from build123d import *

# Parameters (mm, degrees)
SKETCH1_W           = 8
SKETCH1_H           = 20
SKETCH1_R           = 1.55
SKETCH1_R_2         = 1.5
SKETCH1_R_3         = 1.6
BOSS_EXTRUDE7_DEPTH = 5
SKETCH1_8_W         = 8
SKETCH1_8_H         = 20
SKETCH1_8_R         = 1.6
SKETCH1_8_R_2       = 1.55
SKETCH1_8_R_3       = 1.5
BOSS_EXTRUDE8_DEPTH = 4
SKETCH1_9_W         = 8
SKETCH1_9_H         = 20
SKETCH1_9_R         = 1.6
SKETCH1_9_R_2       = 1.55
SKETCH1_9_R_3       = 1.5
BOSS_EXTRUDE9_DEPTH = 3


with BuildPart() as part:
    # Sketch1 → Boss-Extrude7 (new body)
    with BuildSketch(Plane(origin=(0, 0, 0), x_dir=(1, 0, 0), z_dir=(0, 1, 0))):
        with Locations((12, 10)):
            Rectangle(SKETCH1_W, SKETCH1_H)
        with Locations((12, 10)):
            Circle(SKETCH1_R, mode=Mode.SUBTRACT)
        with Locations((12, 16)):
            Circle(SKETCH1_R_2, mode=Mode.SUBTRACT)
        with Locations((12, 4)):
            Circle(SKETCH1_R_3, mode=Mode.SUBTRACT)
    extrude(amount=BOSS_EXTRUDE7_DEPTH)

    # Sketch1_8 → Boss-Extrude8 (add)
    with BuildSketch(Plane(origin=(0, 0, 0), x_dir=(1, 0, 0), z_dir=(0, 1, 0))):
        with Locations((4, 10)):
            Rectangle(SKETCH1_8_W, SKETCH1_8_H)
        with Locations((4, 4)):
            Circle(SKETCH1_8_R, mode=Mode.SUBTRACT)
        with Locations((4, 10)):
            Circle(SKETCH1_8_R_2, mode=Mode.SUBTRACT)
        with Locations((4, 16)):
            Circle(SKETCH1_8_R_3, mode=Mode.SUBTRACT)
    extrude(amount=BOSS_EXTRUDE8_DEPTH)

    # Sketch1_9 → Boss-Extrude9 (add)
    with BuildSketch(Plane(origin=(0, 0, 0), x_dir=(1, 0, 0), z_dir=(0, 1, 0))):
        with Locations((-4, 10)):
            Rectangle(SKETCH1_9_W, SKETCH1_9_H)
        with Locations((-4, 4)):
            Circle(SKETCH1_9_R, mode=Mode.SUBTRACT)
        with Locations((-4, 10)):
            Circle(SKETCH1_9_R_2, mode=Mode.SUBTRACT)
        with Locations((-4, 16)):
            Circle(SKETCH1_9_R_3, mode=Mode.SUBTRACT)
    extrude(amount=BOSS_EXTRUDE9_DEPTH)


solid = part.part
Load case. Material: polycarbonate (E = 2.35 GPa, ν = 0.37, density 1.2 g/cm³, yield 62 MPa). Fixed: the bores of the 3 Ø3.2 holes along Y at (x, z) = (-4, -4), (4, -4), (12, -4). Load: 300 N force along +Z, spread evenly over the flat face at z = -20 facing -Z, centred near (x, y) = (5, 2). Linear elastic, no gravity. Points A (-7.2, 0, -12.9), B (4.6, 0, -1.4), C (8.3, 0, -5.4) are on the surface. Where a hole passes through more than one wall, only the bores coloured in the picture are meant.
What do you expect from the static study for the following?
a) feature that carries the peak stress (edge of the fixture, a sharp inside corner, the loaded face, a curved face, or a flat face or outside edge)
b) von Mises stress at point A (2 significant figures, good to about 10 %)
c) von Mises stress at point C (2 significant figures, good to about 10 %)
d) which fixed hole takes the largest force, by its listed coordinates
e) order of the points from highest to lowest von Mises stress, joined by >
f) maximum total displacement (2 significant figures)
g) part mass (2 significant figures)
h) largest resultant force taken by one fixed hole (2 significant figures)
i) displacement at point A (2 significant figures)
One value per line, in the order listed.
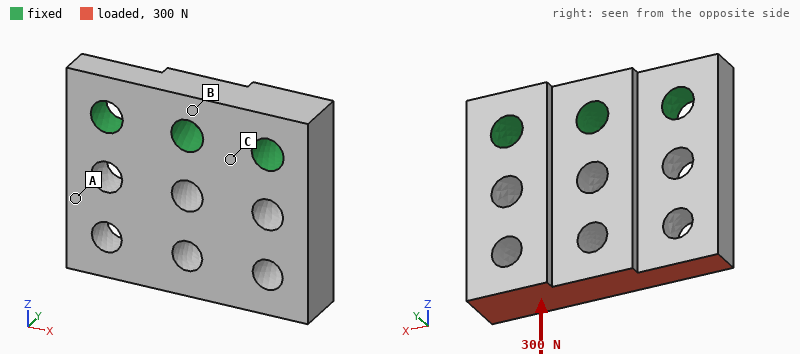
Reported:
a curved face
4.2 MPa
1.8 MPa
(12, -4)
A > C > B
32 µm
2.0 g
130 N
18 µm
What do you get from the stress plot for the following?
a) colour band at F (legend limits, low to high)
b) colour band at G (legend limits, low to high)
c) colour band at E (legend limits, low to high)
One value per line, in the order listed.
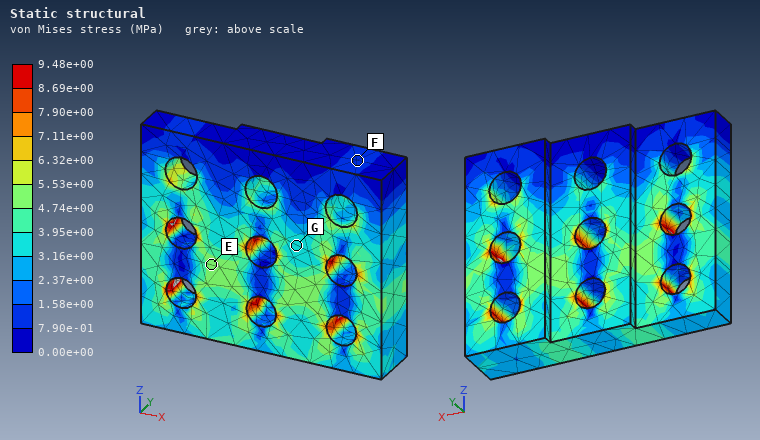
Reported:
7.90e-01 to 1.58e+00 MPa
3.16e+00 to 3.95e+00 MPa
4.74e+00 to 5.53e+00 MPa
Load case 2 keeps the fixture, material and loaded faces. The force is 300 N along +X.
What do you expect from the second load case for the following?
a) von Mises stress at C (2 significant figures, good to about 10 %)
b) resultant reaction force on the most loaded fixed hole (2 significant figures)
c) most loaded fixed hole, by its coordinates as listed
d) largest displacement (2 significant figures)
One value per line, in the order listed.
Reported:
3.9 MPa
300 N
(12, -4)
0.20 mm
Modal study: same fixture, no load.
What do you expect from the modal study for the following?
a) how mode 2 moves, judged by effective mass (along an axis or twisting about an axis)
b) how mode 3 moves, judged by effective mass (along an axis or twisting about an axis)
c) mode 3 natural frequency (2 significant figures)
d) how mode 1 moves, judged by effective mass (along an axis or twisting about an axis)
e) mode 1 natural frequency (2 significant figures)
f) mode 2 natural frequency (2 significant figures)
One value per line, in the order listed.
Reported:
twisting about Z
along X
9400 Hz
along Y
3700 Hz
5600 Hz
